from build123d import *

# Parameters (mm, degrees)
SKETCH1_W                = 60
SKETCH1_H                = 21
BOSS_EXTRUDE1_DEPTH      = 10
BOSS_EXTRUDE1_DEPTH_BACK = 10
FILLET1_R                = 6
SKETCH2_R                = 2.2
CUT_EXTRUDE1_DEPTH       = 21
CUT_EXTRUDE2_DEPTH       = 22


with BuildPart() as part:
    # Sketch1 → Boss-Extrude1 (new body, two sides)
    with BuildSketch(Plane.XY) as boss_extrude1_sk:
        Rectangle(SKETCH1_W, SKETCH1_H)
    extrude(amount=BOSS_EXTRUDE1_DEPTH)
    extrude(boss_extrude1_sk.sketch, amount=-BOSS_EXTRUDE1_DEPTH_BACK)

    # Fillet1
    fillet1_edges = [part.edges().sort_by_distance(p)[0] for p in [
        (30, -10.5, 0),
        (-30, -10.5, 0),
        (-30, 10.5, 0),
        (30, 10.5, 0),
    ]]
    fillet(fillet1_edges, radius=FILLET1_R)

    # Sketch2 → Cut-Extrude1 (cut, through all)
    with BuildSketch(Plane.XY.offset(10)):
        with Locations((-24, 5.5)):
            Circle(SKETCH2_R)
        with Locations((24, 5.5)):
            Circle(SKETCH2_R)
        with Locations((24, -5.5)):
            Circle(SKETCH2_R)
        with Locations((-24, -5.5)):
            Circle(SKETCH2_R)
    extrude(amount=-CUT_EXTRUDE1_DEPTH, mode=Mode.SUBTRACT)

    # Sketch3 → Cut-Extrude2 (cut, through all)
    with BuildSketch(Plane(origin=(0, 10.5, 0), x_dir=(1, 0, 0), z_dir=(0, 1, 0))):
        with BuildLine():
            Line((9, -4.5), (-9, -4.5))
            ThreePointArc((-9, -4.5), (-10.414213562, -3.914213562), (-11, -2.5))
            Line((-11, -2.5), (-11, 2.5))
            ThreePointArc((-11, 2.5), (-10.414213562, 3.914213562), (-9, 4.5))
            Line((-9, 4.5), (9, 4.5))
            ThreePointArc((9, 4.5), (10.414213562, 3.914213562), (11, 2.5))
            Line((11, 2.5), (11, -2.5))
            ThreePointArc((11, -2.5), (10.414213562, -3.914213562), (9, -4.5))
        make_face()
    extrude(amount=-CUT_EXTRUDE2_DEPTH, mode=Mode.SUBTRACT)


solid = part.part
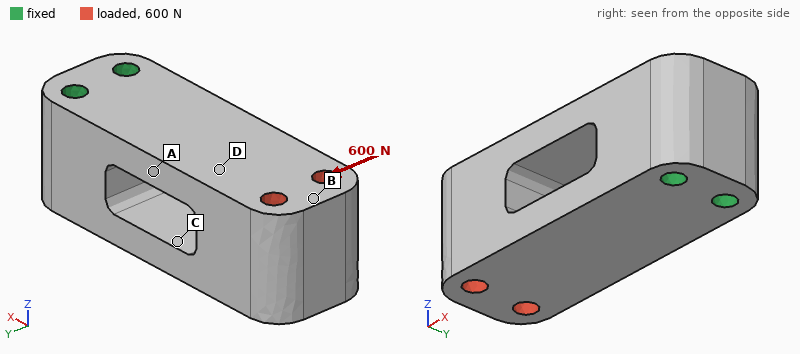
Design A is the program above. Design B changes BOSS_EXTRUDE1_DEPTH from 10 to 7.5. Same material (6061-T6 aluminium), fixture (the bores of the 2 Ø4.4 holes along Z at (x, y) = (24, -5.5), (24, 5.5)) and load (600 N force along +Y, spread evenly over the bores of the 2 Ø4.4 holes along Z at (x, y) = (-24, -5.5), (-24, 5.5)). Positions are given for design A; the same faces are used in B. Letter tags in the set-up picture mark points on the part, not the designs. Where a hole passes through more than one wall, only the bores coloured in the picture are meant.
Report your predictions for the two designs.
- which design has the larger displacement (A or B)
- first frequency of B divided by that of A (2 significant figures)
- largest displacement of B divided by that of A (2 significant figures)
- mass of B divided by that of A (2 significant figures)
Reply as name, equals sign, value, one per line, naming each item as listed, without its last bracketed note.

which design has the larger displacement = B
first frequency of B divided by that of A = 0.86
largest displacement of B divided by that of A = 1.3
mass of B divided by that of A = 0.85
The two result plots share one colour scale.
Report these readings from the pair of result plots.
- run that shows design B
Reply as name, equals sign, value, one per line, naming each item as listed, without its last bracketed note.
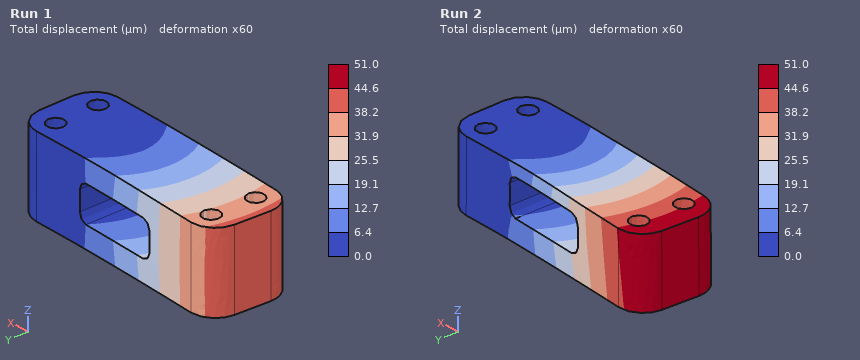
run that shows design B = Run 2
